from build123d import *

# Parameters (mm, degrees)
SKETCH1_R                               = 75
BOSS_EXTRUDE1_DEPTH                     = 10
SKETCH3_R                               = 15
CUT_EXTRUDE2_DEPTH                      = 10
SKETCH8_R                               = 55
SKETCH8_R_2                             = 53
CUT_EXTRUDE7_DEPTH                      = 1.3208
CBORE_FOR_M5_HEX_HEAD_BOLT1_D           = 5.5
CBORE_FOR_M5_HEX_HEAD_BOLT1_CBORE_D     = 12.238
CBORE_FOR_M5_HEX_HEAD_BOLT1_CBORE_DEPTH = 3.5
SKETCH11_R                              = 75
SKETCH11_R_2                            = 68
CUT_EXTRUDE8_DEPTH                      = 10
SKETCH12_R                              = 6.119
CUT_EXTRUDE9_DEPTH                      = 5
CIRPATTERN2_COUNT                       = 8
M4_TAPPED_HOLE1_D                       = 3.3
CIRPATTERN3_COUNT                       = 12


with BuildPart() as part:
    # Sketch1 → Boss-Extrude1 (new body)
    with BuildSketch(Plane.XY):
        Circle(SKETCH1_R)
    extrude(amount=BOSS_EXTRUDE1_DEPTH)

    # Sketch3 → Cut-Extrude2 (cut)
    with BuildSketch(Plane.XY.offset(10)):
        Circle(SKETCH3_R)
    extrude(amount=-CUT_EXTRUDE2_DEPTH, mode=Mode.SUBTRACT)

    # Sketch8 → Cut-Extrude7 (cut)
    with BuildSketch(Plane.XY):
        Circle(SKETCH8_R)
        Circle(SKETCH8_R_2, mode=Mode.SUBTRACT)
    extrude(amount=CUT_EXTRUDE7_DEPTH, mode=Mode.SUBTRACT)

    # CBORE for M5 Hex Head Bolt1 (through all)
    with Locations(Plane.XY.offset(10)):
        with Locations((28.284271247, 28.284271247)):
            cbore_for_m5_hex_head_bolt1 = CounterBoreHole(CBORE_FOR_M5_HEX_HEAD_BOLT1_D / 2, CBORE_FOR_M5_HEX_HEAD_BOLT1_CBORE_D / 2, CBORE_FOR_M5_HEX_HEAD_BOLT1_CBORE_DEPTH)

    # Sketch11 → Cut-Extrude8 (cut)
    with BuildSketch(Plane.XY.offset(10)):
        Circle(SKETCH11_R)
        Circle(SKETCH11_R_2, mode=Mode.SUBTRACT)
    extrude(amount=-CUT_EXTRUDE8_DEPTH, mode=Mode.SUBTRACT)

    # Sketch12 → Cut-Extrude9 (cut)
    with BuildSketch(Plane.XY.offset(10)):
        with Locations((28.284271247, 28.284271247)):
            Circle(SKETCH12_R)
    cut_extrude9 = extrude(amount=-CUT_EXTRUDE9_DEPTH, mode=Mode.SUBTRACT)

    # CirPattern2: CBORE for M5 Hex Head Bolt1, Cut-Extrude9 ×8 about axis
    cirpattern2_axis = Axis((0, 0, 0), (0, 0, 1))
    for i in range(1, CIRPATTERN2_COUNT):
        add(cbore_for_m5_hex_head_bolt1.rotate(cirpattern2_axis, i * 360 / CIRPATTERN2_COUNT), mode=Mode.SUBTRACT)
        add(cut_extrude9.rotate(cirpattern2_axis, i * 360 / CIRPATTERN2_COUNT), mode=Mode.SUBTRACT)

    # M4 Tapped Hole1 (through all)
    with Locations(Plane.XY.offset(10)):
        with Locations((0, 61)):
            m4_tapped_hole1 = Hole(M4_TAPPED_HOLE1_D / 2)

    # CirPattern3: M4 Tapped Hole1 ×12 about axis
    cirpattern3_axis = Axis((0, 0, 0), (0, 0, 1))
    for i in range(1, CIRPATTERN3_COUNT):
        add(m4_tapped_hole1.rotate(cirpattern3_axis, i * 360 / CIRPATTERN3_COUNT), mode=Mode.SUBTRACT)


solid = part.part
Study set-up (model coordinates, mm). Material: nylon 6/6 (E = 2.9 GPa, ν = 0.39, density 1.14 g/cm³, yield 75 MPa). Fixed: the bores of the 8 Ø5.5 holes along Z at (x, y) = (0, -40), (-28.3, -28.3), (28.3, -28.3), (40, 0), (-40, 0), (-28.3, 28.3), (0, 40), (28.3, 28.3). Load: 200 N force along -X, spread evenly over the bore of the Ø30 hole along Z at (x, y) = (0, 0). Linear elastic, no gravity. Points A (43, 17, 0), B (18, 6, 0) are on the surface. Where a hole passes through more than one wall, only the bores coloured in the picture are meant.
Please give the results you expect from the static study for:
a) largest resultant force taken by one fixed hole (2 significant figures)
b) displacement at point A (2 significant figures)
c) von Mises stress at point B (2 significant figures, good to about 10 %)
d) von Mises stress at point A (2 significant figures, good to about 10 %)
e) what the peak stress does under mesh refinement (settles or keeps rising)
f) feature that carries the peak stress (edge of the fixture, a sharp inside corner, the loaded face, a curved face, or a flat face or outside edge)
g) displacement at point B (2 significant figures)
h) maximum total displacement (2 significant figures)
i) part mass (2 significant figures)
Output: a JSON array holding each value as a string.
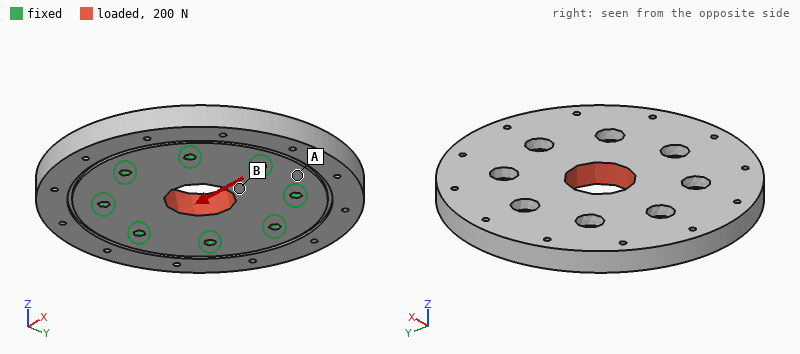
["36 N", "0.79 µm", "0.22 MPa", "0.072 MPa", "keeps rising", "edge of the fixture", "2.0 µm", "3.0 µm", "150 g"]
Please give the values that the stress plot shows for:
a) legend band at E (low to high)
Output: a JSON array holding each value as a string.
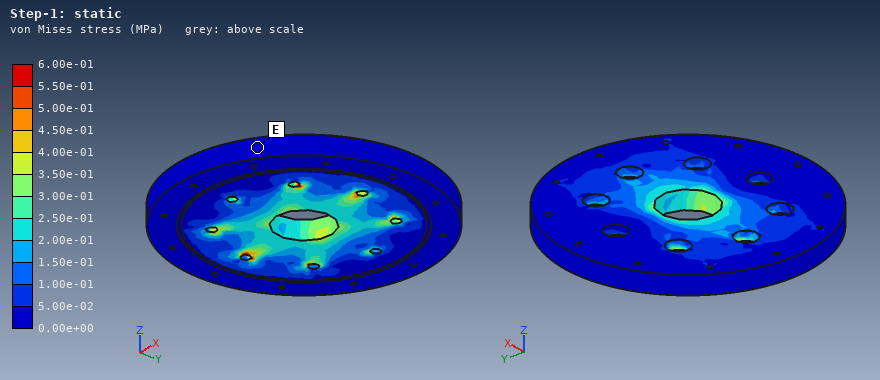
["0.00e+00 to 5.00e-02 MPa"]
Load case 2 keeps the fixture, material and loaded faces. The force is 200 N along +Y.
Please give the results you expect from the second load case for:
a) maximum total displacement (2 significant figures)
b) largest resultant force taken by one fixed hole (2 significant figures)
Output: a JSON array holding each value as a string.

["2.9 µm", "36 N"]
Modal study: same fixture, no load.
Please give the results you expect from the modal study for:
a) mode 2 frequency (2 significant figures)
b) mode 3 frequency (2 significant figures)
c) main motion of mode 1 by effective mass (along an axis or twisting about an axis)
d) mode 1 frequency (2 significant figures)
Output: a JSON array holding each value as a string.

["2000 Hz", "2000 Hz", "along Z", "1800 Hz"]
